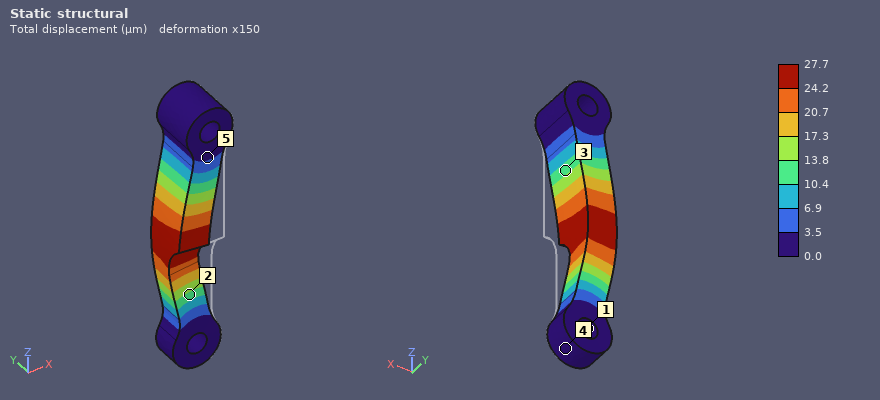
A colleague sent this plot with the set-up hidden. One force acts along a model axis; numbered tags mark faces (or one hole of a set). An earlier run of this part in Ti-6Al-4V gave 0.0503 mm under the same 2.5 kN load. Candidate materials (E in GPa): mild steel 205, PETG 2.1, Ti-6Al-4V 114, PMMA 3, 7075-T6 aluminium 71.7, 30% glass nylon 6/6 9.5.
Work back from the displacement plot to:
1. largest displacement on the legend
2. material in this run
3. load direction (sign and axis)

27.7 µm
mild steel
-X
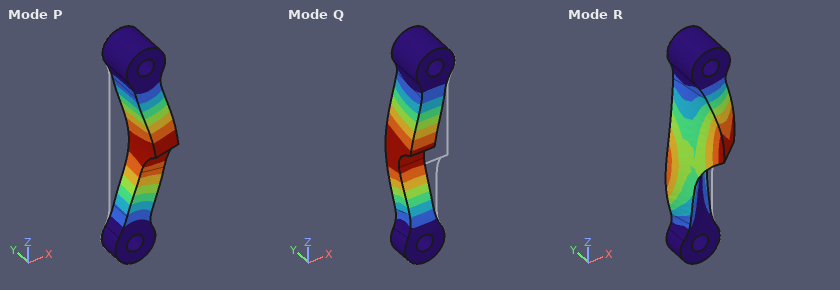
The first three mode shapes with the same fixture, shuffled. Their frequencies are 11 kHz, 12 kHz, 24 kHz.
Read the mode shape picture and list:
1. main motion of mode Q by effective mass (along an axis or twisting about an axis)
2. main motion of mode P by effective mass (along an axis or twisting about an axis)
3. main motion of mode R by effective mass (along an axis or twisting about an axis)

along Y
along X
twisting about Z
